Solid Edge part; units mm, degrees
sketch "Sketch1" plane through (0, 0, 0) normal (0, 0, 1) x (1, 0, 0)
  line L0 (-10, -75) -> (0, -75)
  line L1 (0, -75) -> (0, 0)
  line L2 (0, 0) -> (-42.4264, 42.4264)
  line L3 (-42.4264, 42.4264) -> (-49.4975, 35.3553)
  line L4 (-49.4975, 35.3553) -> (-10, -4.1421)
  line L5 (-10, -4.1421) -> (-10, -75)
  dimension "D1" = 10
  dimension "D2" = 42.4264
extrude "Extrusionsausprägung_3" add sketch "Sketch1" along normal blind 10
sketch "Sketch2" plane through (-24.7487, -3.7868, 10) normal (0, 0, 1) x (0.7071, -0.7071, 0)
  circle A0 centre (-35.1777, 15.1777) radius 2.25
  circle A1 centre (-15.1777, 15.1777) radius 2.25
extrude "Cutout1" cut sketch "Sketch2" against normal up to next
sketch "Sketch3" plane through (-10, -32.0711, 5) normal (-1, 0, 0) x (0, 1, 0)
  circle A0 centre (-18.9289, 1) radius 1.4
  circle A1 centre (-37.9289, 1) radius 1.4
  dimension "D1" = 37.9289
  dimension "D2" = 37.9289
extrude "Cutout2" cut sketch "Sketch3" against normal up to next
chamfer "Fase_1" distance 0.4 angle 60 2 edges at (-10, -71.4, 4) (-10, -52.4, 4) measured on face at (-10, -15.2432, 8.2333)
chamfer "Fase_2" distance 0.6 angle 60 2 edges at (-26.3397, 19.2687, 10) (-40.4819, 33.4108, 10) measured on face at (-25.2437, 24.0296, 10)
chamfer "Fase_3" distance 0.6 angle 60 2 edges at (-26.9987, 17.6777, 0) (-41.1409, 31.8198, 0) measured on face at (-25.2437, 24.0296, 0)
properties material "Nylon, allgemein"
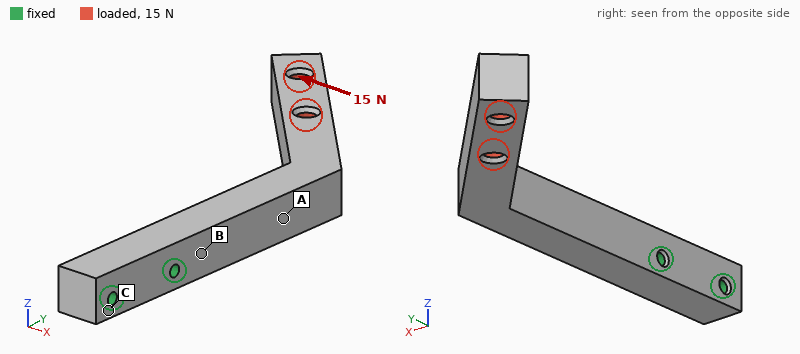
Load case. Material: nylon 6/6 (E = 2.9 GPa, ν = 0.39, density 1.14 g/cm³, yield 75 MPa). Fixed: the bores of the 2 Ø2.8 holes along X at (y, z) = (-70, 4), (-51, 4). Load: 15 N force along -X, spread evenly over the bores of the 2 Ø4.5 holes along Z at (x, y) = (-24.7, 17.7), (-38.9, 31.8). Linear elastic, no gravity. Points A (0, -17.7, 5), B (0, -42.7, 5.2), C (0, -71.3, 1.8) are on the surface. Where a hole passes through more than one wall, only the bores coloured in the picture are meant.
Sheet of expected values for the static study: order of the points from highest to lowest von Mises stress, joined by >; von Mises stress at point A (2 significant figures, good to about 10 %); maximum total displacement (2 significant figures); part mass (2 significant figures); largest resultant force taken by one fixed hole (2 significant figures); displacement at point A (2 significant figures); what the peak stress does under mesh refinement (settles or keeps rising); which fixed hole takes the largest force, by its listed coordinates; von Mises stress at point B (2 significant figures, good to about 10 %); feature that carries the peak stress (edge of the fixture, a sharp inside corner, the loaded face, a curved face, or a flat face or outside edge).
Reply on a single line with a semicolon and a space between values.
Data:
B > A > C; 3.8 MPa; 1.5 mm; 14 g; 27 N; 0.25 mm; keeps rising; (-51, 4); 6.2 MPa; edge of the fixture
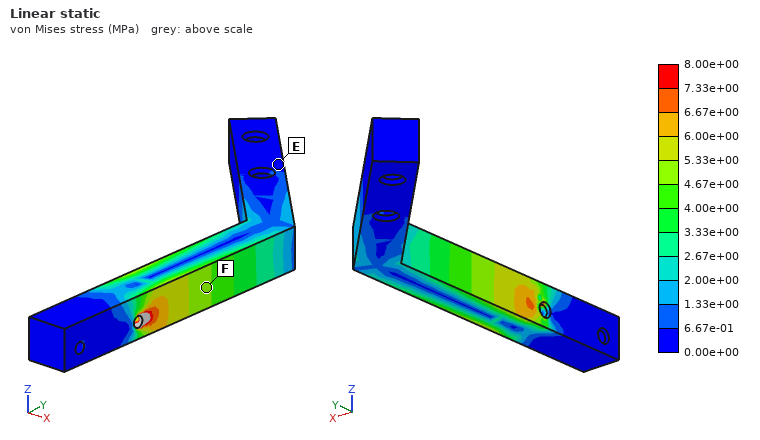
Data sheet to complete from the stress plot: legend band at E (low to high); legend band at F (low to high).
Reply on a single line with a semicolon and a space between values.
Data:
0.00e+00 to 6.67e-01 MPa; 4.67e+00 to 5.33e+00 MPa
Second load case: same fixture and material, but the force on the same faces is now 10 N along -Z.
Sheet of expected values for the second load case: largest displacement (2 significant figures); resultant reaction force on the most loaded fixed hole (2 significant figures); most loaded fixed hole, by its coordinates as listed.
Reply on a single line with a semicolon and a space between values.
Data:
1.3 mm; 40 N; (-51, 4)
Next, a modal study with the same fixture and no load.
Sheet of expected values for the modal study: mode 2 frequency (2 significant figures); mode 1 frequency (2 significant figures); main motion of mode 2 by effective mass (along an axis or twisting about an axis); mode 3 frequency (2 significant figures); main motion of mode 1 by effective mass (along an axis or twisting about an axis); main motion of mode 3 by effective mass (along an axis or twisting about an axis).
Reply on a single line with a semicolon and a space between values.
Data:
250 Hz; 230 Hz; along X; 940 Hz; along Z; along Z
